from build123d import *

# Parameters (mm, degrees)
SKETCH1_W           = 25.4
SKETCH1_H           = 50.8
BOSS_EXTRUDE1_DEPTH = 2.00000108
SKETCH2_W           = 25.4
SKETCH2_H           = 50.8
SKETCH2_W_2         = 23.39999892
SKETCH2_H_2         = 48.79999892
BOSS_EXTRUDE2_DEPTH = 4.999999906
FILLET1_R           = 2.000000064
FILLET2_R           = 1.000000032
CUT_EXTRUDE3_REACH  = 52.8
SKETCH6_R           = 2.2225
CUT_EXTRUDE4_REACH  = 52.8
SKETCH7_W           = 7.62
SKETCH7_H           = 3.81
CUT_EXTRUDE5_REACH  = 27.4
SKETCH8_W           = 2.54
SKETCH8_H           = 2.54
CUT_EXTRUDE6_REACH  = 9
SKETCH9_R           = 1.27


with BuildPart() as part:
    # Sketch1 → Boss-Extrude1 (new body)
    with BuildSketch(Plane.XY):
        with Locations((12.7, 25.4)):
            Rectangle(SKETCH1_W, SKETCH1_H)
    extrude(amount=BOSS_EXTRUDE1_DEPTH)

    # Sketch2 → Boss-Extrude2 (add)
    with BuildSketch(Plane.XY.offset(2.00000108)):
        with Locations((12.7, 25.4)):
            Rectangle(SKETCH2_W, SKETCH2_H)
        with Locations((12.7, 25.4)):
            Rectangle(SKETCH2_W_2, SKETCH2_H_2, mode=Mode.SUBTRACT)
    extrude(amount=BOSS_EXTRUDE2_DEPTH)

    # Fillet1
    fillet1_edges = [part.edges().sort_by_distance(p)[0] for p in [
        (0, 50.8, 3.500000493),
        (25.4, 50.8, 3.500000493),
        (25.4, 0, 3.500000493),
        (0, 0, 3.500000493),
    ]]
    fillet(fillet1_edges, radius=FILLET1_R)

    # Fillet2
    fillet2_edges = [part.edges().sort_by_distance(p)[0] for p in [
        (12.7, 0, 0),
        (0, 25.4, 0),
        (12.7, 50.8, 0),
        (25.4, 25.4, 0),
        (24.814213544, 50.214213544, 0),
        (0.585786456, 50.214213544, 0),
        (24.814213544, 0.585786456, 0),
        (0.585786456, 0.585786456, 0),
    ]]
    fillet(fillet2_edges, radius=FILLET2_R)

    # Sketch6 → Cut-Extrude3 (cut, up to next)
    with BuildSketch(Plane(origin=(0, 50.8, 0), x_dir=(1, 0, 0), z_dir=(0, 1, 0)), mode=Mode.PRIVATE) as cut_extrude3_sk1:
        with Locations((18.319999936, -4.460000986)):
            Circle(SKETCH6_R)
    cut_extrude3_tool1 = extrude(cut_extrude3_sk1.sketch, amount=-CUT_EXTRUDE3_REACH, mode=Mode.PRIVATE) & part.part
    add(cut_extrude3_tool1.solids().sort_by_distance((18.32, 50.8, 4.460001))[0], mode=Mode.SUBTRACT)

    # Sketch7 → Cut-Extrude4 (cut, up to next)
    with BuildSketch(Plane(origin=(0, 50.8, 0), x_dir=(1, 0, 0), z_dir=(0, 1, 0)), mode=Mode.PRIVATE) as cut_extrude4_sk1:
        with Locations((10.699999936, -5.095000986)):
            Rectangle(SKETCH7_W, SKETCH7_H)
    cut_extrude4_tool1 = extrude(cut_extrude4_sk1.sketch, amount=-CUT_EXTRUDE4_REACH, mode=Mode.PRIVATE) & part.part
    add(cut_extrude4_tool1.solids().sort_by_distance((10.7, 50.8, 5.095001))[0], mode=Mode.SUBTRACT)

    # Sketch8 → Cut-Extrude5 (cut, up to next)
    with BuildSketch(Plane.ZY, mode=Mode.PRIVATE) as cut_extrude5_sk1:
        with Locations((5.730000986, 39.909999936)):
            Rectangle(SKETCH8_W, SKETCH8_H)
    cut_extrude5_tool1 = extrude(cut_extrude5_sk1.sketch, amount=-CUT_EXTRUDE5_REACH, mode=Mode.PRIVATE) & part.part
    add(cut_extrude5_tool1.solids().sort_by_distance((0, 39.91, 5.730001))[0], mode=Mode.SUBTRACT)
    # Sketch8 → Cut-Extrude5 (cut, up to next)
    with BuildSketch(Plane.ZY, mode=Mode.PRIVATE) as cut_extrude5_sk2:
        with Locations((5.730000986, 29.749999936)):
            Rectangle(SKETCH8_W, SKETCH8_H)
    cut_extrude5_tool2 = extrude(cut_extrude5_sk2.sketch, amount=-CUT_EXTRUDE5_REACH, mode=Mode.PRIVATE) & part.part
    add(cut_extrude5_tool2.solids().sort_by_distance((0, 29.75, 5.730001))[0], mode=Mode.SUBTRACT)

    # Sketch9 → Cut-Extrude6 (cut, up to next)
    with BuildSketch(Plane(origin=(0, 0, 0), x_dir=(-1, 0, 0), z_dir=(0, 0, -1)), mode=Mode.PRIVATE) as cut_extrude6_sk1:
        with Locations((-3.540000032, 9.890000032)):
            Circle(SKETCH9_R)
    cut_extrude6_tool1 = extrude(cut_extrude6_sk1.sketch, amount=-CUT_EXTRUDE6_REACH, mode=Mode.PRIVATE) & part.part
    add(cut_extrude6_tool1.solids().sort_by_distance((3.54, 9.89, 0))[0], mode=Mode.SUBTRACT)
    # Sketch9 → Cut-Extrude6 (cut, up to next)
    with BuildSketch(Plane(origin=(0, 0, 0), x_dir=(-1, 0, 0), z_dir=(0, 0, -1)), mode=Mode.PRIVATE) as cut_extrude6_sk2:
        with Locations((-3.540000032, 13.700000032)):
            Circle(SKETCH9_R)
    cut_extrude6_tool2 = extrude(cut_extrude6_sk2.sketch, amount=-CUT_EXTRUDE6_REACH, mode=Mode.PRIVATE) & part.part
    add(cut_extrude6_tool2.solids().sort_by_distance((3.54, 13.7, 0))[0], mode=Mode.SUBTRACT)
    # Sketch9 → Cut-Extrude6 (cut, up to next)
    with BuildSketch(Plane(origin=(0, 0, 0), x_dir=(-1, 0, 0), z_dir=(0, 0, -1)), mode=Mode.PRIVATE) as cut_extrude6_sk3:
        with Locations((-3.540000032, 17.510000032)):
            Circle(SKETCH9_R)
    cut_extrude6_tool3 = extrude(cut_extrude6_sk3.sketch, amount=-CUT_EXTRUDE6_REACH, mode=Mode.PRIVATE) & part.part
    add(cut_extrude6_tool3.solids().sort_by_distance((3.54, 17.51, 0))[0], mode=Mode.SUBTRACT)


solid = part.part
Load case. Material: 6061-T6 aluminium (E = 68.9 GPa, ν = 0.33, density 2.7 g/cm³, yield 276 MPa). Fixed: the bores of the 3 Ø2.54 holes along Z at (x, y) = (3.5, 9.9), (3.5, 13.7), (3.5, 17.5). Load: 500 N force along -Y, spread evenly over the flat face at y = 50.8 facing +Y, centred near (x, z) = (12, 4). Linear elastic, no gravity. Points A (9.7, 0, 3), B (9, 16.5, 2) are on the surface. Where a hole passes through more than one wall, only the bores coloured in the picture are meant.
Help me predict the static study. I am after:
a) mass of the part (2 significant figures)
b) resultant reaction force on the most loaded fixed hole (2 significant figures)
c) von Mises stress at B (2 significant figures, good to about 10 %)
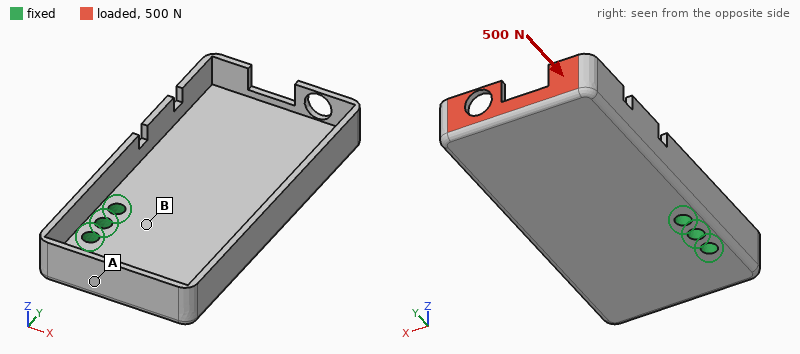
8.6 g
480 N
54 MPa
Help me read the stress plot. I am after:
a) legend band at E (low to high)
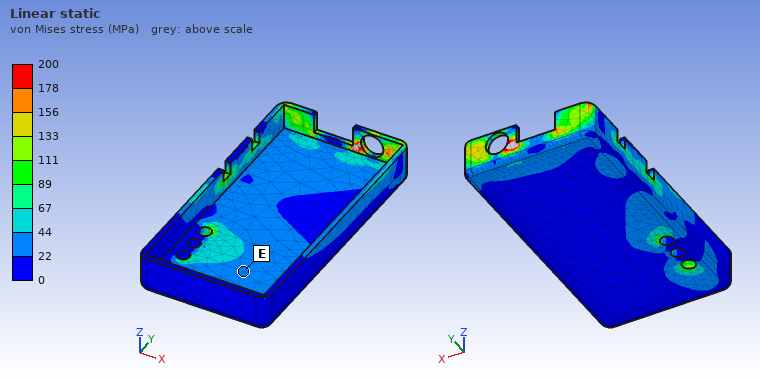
22 to 44 MPa
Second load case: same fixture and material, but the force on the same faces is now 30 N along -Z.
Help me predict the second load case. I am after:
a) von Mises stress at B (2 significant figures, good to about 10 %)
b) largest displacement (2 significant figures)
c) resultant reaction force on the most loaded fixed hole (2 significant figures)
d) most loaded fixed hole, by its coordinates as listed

27 MPa
0.20 mm
110 N
(3.5, 17.5)
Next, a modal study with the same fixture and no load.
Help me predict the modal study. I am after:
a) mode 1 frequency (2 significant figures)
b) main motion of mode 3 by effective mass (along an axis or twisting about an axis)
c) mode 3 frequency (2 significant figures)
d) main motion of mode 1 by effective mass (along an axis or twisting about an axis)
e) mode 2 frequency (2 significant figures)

1500 Hz
along Z
4300 Hz
along Z
3000 Hz
